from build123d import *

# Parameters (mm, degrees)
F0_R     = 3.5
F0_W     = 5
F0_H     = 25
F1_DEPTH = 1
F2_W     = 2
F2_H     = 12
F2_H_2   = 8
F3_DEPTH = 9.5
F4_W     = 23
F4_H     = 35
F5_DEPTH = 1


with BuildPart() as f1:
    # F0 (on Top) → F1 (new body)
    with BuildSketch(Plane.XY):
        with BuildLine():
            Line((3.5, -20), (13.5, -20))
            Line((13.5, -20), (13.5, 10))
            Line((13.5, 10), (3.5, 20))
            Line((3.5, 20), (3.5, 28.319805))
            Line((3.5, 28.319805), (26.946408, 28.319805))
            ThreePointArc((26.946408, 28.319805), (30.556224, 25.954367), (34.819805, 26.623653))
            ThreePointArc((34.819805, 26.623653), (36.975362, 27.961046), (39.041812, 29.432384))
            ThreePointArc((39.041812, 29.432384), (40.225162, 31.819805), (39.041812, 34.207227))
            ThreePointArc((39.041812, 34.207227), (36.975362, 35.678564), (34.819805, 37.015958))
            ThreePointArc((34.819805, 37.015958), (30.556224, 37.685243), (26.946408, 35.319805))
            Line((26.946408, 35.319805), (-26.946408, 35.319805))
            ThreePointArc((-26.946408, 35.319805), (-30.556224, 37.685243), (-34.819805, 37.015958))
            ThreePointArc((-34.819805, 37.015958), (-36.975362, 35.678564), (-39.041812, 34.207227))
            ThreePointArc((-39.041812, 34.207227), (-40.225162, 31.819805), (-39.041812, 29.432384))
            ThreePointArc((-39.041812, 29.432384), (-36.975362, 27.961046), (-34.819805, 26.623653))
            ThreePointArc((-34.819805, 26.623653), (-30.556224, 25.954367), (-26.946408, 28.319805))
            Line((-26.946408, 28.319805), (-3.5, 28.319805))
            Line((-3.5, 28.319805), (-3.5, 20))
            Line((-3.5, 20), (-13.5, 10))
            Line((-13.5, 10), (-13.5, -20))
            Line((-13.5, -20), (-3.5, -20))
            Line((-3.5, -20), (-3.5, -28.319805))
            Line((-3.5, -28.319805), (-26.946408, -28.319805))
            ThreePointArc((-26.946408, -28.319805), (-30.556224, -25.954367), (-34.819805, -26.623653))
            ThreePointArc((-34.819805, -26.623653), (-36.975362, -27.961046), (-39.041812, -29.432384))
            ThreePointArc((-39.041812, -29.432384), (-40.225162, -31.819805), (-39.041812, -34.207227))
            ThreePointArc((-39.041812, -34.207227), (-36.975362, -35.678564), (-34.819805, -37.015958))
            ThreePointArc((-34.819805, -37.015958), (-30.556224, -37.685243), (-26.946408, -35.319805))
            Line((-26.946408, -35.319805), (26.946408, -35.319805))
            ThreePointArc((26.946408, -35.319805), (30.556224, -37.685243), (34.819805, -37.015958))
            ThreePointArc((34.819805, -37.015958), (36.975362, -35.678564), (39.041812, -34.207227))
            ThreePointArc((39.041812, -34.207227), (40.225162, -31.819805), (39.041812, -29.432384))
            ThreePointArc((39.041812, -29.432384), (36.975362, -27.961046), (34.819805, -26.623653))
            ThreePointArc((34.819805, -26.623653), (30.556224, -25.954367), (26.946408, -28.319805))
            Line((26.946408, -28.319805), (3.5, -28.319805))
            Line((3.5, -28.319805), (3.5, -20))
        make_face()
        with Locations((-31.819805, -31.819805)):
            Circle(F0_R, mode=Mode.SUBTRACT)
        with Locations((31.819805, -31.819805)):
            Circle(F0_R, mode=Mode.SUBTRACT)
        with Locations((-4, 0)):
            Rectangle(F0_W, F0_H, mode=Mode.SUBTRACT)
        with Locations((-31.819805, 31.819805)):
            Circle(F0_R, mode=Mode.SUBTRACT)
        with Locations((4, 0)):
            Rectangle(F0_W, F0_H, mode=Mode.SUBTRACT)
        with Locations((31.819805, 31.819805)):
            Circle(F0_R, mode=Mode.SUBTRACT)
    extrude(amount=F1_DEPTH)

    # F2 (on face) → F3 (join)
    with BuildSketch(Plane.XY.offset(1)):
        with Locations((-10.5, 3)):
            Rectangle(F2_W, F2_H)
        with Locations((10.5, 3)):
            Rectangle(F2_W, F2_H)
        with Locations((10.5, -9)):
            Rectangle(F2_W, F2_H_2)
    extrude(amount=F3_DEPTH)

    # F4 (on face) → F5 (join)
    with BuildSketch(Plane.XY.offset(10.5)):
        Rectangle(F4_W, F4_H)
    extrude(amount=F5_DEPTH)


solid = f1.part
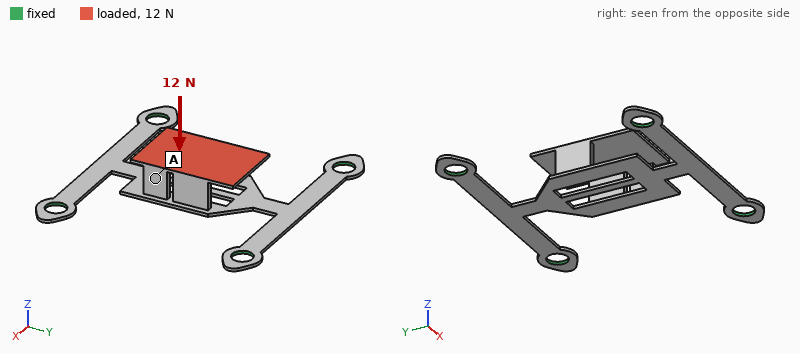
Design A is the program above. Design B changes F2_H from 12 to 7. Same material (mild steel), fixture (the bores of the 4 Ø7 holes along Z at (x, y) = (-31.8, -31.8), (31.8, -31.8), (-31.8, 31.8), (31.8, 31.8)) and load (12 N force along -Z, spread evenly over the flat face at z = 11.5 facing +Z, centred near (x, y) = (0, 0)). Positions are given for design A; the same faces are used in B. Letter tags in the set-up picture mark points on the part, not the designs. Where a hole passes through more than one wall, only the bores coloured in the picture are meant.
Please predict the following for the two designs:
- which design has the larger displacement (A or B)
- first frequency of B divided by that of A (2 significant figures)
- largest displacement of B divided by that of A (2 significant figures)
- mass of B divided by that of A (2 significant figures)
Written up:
B
1.0
1.1
0.94
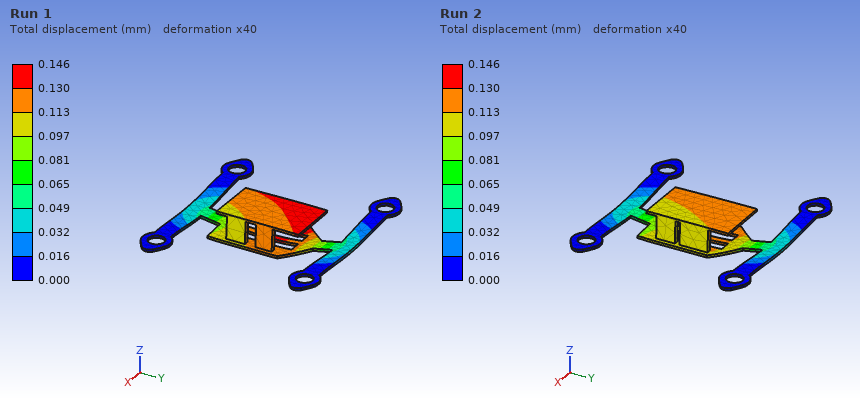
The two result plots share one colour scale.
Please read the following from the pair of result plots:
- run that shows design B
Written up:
Run 1
